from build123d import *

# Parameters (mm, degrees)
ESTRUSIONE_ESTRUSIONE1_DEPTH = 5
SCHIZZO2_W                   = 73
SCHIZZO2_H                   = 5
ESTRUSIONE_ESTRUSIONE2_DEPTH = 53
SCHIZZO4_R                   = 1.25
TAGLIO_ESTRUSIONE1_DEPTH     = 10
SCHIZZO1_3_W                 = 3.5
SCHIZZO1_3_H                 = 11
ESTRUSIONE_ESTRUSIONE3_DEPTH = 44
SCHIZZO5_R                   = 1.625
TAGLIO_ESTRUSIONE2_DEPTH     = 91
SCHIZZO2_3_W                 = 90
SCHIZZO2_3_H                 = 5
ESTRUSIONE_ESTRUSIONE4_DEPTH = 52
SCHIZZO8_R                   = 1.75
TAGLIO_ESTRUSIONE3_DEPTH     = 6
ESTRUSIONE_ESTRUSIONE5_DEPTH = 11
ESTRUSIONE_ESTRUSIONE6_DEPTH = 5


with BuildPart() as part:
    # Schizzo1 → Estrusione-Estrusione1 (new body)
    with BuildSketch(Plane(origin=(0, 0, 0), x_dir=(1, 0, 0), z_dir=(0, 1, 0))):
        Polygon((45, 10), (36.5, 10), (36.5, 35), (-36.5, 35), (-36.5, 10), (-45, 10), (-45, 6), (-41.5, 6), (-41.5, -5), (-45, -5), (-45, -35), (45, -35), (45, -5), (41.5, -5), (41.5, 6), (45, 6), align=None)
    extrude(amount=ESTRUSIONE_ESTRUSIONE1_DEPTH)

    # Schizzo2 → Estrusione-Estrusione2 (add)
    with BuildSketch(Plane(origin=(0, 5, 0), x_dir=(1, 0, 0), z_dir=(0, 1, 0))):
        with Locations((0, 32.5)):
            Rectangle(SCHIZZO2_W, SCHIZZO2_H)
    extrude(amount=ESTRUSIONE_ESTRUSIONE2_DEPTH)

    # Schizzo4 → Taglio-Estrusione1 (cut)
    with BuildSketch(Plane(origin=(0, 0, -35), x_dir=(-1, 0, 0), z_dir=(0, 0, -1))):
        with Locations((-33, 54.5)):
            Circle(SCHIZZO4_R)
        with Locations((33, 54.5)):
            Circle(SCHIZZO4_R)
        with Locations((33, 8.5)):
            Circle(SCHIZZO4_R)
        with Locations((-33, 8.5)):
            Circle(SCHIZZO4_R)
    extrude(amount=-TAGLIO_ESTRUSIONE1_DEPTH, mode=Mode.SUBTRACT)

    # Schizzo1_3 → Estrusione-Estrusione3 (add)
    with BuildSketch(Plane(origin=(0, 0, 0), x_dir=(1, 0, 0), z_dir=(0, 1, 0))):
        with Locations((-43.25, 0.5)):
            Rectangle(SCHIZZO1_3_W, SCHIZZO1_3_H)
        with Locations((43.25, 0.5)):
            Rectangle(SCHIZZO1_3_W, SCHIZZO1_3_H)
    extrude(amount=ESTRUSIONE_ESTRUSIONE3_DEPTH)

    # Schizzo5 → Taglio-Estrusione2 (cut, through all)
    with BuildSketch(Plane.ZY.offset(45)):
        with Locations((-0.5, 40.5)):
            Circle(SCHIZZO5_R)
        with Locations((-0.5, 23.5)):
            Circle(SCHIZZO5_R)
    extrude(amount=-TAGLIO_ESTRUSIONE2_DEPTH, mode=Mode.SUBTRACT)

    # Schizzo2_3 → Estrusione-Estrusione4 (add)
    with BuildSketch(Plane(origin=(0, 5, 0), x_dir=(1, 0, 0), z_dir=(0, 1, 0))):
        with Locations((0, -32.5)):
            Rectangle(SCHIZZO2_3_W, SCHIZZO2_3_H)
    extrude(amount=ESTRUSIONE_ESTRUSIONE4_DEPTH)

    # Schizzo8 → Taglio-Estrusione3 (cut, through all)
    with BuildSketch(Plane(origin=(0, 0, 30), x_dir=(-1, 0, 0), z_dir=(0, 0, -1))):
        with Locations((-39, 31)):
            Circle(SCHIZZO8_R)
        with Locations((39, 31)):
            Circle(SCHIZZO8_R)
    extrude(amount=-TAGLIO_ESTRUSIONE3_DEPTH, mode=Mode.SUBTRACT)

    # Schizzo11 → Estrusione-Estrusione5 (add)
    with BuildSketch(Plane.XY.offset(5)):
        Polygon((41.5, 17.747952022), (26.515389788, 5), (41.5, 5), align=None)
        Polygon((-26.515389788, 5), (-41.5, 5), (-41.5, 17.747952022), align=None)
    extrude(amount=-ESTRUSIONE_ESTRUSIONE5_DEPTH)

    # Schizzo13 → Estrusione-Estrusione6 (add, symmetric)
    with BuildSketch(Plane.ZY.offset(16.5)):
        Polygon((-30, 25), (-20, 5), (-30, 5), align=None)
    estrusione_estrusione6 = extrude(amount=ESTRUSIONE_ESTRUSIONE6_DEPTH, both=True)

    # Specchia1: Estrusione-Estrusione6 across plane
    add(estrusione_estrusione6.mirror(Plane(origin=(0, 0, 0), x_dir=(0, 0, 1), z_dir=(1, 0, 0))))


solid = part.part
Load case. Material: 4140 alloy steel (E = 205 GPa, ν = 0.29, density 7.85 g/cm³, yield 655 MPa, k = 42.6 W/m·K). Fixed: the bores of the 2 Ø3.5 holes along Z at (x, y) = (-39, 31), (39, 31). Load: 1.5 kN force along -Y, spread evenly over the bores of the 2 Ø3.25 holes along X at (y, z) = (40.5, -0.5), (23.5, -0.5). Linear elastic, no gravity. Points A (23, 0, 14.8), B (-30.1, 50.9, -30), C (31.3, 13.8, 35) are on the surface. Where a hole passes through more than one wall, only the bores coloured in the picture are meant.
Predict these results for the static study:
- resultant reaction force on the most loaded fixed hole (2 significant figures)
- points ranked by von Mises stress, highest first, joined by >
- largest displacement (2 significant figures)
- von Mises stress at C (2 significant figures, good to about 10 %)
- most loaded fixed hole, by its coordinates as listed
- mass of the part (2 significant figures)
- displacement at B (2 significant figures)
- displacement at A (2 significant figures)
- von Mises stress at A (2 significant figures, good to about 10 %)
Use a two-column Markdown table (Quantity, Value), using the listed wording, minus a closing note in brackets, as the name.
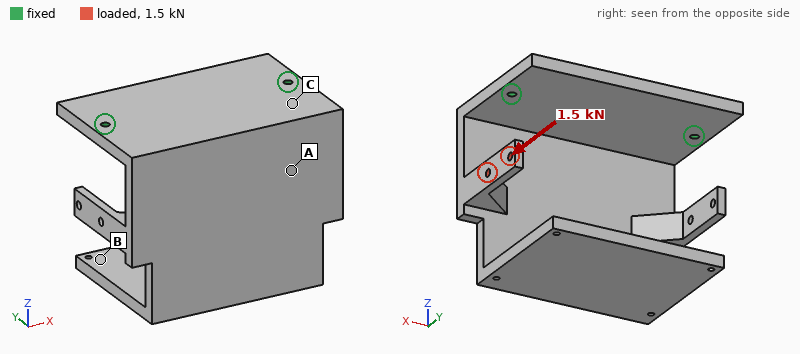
| Quantity | Value |
|---|---|
| resultant reaction force on the most loaded fixed hole | 1.6 kN |
| points ranked by von Mises stress, highest first, joined by > | C > A > B |
| largest displacement | 1.2 mm |
| von Mises stress at C | 170 MPa |
| most loaded fixed hole, by its coordinates as listed | (39, 31) |
| mass of the part | 620 g |
| displacement at B | 0.83 mm |
| displacement at A | 0.32 mm |
| von Mises stress at A | 100 MPa |
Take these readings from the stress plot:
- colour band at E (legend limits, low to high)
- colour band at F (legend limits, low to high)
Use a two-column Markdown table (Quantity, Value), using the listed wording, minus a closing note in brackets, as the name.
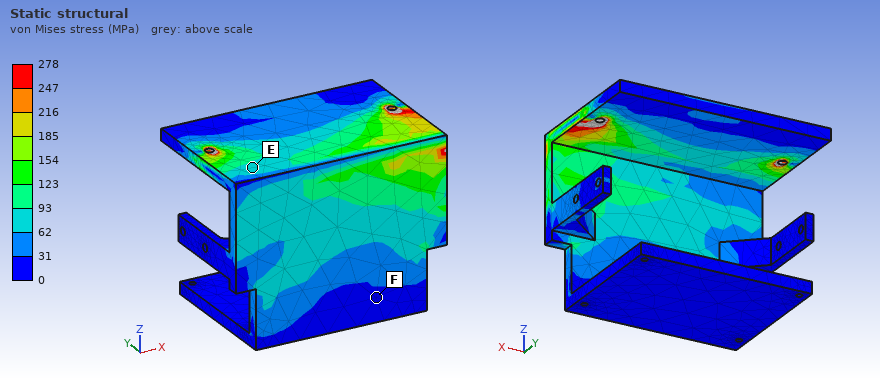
| Quantity | Value |
|---|---|
| colour band at E | 62 to 93 MPa |
| colour band at F | 0 to 31 MPa |
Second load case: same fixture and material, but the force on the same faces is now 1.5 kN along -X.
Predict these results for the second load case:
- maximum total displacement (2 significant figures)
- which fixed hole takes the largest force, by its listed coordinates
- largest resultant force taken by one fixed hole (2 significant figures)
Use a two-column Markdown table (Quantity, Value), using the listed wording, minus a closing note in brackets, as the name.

| Quantity | Value |
|---|---|
| maximum total displacement | 1.2 mm |
| which fixed hole takes the largest force, by its listed coordinates | (39, 31) |
| largest resultant force taken by one fixed hole | 1.1 kN |
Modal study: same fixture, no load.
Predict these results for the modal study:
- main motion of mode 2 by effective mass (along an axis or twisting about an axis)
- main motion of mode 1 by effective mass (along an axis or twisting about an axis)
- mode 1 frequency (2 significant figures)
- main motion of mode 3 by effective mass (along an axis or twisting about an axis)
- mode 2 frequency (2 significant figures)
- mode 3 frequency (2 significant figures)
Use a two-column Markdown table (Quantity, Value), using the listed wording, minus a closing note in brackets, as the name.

| Quantity | Value |
|---|---|
| main motion of mode 2 by effective mass | along X |
| main motion of mode 1 by effective mass | along Y |
| mode 1 frequency | 280 Hz |
| main motion of mode 3 by effective mass | along Z |
| mode 2 frequency | 580 Hz |
| mode 3 frequency | 840 Hz |
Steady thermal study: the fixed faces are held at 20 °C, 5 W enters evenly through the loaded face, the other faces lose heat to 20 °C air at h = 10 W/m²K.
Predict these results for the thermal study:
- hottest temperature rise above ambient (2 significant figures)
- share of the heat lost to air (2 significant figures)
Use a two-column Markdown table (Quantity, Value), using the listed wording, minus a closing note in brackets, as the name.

| Quantity | Value |
|---|---|
| hottest temperature rise above ambient | 82 K |
| share of the heat lost to air | 53 % |
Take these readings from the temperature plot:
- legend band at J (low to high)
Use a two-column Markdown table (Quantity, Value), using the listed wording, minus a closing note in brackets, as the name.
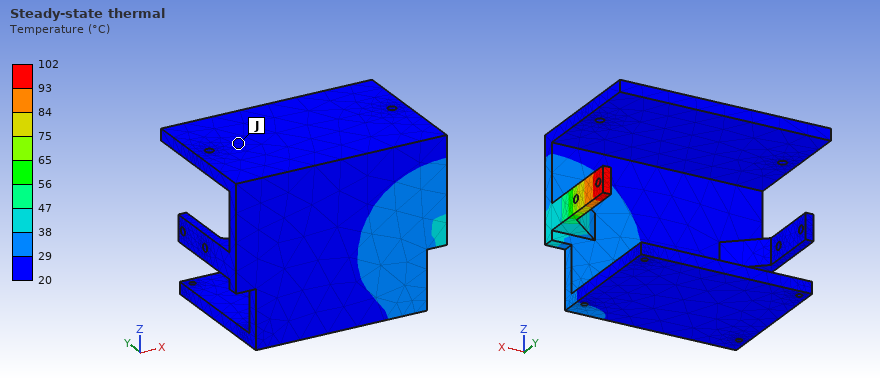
| Quantity | Value |
|---|---|
| legend band at J | 20 to 29 °C |
